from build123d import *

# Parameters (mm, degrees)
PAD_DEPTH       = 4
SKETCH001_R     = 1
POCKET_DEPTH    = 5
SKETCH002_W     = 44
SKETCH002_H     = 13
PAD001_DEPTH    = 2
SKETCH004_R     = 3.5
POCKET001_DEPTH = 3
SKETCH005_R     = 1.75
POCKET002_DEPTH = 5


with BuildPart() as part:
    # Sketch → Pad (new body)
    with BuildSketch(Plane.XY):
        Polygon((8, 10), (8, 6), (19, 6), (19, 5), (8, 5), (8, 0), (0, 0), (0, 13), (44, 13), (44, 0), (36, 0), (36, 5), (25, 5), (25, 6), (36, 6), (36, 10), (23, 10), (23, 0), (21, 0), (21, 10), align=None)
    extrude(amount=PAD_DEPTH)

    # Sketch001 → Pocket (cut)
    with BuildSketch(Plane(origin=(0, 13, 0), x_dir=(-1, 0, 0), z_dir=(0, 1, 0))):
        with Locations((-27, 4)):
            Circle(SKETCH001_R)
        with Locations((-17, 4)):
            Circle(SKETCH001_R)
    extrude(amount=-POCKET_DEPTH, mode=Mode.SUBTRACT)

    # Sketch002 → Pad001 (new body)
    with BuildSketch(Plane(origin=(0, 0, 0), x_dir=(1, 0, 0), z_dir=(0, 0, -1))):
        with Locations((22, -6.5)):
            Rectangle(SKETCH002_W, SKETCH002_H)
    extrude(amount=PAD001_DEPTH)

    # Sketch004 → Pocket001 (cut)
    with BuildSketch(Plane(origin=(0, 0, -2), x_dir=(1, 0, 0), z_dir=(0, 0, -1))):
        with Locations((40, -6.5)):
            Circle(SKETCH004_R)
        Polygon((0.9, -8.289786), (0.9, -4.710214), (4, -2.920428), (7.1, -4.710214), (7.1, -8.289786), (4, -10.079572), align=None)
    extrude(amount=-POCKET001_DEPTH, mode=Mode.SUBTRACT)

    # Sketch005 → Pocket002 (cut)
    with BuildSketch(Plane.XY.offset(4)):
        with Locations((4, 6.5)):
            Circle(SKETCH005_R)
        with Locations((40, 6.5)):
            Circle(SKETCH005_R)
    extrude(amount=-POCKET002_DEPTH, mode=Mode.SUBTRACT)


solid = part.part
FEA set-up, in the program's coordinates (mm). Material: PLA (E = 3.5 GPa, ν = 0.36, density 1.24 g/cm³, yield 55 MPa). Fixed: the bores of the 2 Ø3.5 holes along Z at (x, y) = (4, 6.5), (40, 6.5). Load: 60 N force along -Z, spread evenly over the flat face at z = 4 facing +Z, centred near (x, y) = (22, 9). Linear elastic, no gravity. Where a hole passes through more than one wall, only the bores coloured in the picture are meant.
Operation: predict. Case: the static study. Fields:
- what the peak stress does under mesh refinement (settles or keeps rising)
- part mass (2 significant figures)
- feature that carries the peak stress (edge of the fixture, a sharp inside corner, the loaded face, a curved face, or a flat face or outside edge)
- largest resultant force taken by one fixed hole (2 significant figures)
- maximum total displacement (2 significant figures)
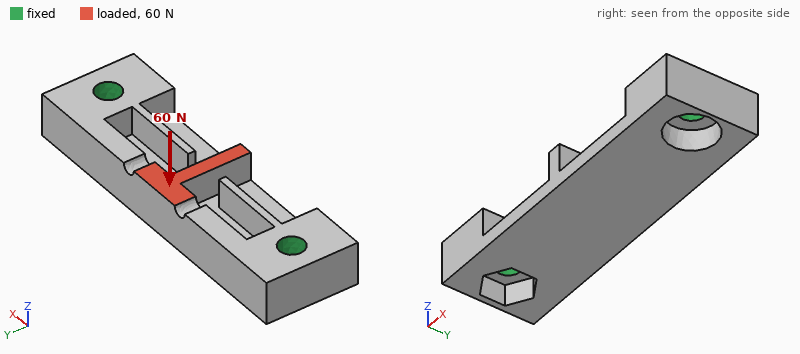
keeps rising
2.7 g
edge of the fixture
53 N
82 µm
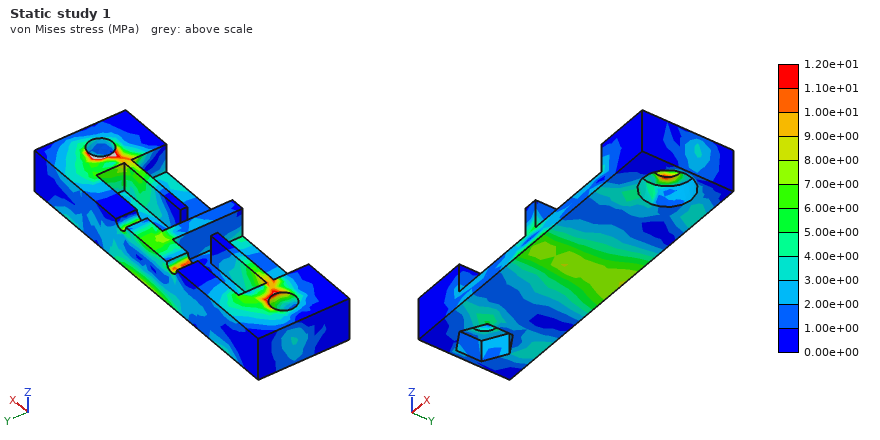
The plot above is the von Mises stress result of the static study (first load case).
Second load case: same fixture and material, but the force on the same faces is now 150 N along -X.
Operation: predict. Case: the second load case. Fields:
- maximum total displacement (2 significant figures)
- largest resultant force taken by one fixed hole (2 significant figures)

0.18 mm
78 N
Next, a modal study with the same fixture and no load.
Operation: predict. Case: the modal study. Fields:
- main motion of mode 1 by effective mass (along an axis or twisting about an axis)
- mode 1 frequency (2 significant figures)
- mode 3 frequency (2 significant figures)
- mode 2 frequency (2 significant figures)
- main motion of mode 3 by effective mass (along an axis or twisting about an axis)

along Z
4900 Hz
6700 Hz
5900 Hz
along Y
